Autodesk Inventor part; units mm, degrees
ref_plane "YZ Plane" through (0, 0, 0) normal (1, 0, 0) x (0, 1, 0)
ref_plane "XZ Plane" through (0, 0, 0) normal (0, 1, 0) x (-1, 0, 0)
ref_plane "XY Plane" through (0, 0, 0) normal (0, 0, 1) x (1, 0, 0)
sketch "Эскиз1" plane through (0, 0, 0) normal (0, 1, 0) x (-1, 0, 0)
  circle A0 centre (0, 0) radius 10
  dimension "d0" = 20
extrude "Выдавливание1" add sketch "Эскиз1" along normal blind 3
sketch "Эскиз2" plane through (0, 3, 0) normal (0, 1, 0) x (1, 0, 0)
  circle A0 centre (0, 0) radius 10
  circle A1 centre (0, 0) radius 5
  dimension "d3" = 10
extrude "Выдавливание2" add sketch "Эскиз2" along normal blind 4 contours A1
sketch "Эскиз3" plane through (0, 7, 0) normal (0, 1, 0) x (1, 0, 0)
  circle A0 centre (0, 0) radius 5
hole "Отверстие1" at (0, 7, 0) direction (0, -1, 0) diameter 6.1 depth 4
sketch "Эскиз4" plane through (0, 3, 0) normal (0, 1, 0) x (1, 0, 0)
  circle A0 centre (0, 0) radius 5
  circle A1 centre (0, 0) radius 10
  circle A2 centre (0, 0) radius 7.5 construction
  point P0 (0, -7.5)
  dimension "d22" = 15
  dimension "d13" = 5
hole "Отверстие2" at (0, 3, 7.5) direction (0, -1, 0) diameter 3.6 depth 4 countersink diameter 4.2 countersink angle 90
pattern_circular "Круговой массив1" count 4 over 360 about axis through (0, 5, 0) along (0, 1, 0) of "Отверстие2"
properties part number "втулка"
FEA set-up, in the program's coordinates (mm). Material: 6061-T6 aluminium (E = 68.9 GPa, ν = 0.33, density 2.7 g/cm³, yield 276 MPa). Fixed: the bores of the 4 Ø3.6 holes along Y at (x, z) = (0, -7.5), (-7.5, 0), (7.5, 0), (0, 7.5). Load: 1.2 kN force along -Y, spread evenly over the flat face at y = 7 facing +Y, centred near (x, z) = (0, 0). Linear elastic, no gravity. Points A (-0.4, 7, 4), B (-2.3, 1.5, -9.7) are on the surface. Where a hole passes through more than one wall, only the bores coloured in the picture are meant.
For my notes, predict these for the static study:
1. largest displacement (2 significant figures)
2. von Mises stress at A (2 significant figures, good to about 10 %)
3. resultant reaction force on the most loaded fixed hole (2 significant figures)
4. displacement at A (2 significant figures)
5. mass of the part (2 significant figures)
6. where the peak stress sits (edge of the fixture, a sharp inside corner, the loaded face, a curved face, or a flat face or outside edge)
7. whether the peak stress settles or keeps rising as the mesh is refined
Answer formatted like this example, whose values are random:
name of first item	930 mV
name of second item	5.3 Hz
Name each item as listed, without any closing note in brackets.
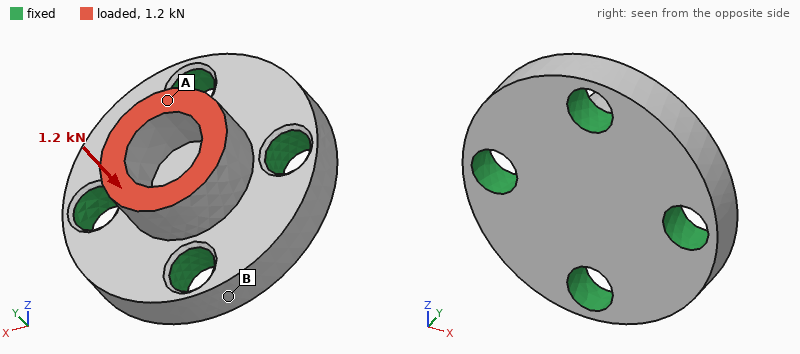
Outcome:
largest displacement	3.3 µm
von Mises stress at A	25 MPa
resultant reaction force on the most loaded fixed hole	320 N
displacement at A	3.1 µm
mass of the part	2.7 g
where the peak stress sits	edge of the fixture
whether the peak stress settles or keeps rising as the mesh is refined	keeps rising
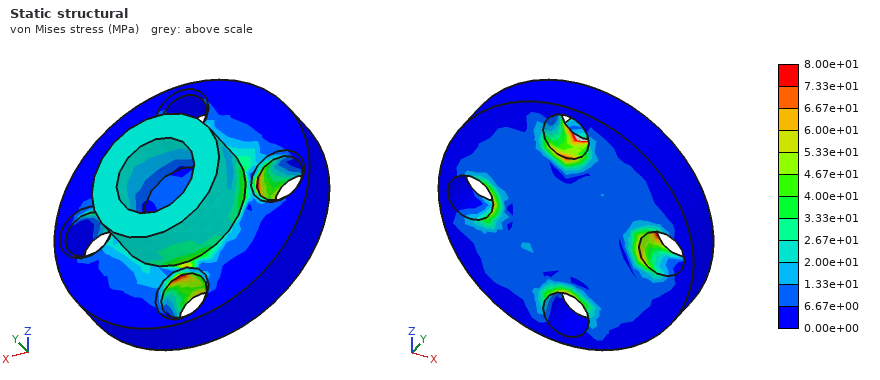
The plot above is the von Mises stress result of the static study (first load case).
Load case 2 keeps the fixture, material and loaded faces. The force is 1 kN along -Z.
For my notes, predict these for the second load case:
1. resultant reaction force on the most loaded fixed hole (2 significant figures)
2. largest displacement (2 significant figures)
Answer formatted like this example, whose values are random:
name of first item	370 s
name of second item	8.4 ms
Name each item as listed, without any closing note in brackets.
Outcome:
resultant reaction force on the most loaded fixed hole	520 N
largest displacement	13 µm
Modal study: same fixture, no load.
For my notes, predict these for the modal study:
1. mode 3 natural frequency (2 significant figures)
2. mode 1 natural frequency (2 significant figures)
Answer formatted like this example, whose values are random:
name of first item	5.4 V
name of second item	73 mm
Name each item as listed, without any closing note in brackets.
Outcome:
mode 3 natural frequency	100 kHz
mode 1 natural frequency	98 kHz
